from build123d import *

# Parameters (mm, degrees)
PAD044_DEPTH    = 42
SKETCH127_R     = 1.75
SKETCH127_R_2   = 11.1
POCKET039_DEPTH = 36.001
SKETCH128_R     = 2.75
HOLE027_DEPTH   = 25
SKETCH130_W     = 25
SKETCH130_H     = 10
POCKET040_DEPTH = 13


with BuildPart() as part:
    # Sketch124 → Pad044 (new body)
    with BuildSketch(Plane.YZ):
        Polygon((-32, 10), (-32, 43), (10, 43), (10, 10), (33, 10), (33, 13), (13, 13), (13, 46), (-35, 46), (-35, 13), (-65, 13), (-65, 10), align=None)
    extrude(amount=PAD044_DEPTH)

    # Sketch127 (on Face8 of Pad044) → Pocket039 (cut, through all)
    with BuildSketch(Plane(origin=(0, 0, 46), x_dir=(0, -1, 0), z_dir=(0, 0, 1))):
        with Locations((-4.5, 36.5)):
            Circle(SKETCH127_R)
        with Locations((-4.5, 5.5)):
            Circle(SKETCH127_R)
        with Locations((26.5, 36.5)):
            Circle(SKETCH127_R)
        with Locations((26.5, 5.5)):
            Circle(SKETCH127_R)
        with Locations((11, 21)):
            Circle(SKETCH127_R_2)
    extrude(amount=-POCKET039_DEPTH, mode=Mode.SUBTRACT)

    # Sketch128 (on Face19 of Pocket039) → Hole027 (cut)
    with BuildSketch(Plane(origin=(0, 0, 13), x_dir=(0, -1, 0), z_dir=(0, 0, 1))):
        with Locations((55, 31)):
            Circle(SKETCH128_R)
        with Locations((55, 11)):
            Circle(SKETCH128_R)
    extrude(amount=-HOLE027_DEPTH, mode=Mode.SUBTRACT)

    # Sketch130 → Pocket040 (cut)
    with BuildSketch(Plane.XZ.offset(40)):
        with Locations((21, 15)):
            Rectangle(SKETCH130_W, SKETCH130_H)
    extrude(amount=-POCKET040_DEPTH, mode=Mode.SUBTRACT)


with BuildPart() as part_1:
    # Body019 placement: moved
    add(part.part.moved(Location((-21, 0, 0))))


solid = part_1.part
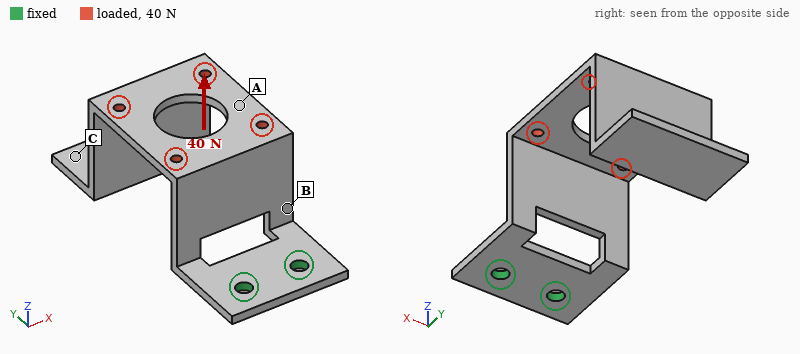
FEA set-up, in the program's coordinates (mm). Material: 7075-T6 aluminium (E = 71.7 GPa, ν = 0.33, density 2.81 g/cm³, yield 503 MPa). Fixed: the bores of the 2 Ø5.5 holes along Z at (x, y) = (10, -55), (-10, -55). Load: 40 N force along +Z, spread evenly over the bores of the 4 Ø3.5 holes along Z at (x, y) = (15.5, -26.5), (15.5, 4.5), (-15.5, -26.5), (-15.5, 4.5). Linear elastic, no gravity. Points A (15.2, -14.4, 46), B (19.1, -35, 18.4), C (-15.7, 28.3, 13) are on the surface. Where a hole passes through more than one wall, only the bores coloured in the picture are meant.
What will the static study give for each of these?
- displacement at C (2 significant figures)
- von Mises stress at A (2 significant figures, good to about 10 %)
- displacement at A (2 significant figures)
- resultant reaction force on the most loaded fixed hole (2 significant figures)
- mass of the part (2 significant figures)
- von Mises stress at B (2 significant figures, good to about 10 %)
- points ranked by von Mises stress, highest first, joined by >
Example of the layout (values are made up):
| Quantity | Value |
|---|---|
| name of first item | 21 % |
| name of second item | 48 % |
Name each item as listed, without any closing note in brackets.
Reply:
| Quantity | Value |
|---|---|
| displacement at C | 1.0 mm |
| von Mises stress at A | 12 MPa |
| displacement at A | 0.49 mm |
| resultant reaction force on the most loaded fixed hole | 20 N |
| mass of the part | 51 g |
| von Mises stress at B | 33 MPa |
| points ranked by von Mises stress, highest first, joined by > | B > A > C |
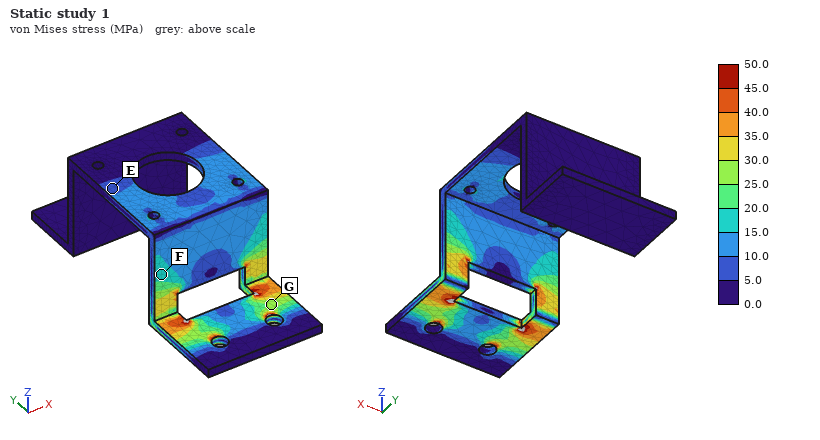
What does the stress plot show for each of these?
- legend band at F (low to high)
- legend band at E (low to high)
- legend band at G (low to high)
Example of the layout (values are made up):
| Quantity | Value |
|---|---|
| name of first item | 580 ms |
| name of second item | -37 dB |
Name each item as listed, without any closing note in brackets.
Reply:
| Quantity | Value |
|---|---|
| legend band at F | 15.0 to 20.0 MPa |
| legend band at E | 5.0 to 10.0 MPa |
| legend band at G | 25.0 to 30.0 MPa |
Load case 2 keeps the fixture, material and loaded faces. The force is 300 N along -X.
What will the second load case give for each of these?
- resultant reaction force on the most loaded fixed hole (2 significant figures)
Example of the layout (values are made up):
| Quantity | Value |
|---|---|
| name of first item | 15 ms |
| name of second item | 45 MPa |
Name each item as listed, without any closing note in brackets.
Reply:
| Quantity | Value |
|---|---|
| resultant reaction force on the most loaded fixed hole | 630 N |
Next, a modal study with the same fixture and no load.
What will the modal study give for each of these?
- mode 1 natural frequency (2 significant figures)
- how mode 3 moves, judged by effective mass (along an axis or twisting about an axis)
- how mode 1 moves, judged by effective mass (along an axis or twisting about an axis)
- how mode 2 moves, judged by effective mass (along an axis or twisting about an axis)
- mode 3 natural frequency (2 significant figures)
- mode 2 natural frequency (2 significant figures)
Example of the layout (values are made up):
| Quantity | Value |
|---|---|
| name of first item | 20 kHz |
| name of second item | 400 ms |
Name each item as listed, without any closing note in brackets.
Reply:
| Quantity | Value |
|---|---|
| mode 1 natural frequency | 150 Hz |
| how mode 3 moves, judged by effective mass | along Y |
| how mode 1 moves, judged by effective mass | along Z |
| how mode 2 moves, judged by effective mass | along X |
| mode 3 natural frequency | 380 Hz |
| mode 2 natural frequency | 310 Hz |
